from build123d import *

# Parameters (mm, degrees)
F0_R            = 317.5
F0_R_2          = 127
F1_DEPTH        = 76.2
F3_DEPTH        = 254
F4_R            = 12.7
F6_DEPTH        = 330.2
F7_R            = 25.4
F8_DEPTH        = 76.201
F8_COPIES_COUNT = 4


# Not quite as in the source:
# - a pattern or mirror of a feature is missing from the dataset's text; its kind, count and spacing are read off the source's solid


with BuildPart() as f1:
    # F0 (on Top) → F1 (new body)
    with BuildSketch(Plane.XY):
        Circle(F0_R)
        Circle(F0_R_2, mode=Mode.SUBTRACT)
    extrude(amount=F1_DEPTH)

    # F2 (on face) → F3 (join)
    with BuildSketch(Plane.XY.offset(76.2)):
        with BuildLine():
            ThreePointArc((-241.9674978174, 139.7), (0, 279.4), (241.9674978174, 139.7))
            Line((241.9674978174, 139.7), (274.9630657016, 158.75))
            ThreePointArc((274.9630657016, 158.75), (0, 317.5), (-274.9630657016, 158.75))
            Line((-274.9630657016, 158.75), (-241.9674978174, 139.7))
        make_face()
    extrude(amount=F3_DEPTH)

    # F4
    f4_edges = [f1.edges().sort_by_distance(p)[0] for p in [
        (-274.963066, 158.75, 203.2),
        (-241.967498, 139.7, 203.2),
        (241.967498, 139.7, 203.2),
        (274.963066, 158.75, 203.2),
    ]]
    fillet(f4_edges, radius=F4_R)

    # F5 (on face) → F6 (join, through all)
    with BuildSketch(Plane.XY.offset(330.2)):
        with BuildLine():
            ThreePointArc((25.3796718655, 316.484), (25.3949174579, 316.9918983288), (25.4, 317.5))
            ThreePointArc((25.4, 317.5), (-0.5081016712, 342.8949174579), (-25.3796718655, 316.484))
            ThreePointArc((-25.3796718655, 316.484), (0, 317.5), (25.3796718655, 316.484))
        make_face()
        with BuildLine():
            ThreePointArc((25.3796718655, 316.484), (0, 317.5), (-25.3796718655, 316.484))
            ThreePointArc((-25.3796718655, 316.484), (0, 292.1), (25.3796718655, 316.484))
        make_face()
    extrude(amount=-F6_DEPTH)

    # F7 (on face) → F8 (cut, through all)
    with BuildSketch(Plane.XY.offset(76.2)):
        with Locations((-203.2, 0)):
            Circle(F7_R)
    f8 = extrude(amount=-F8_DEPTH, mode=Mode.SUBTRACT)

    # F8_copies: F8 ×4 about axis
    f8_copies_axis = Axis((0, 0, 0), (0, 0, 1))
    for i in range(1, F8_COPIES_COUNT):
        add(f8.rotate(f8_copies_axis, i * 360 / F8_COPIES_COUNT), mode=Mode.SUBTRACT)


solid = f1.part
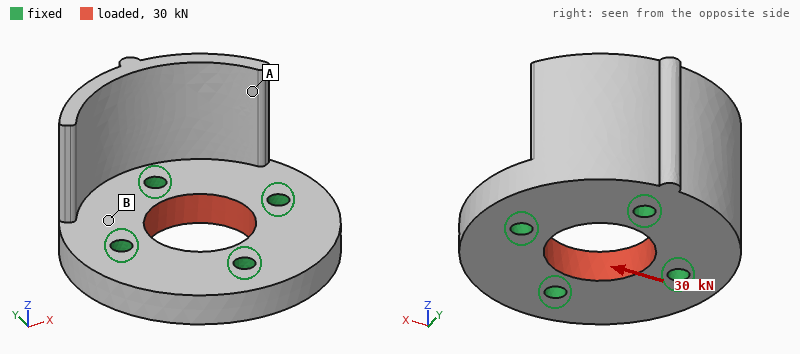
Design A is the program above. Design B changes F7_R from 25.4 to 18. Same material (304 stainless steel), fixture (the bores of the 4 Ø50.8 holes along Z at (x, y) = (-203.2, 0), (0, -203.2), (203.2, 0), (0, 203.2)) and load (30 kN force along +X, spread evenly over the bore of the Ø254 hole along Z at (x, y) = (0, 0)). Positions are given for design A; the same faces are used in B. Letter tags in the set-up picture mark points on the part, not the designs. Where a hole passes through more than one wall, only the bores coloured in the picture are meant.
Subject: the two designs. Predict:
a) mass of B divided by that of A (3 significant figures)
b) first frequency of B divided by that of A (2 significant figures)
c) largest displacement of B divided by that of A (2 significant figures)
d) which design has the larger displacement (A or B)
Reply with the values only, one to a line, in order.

1.01
0.97
1.1
B
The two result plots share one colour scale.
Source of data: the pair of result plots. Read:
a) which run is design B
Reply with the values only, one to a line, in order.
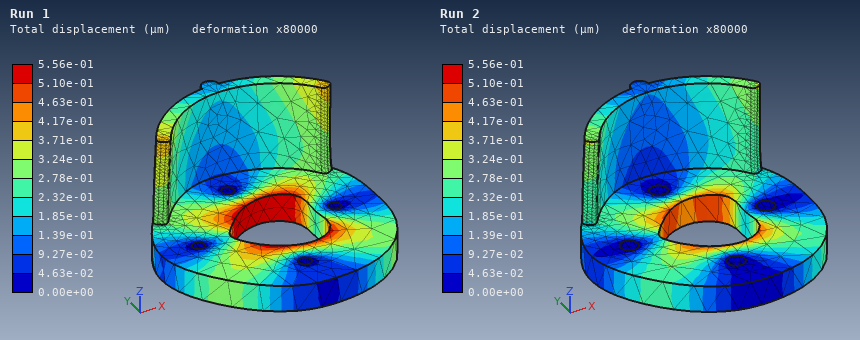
Run 1
